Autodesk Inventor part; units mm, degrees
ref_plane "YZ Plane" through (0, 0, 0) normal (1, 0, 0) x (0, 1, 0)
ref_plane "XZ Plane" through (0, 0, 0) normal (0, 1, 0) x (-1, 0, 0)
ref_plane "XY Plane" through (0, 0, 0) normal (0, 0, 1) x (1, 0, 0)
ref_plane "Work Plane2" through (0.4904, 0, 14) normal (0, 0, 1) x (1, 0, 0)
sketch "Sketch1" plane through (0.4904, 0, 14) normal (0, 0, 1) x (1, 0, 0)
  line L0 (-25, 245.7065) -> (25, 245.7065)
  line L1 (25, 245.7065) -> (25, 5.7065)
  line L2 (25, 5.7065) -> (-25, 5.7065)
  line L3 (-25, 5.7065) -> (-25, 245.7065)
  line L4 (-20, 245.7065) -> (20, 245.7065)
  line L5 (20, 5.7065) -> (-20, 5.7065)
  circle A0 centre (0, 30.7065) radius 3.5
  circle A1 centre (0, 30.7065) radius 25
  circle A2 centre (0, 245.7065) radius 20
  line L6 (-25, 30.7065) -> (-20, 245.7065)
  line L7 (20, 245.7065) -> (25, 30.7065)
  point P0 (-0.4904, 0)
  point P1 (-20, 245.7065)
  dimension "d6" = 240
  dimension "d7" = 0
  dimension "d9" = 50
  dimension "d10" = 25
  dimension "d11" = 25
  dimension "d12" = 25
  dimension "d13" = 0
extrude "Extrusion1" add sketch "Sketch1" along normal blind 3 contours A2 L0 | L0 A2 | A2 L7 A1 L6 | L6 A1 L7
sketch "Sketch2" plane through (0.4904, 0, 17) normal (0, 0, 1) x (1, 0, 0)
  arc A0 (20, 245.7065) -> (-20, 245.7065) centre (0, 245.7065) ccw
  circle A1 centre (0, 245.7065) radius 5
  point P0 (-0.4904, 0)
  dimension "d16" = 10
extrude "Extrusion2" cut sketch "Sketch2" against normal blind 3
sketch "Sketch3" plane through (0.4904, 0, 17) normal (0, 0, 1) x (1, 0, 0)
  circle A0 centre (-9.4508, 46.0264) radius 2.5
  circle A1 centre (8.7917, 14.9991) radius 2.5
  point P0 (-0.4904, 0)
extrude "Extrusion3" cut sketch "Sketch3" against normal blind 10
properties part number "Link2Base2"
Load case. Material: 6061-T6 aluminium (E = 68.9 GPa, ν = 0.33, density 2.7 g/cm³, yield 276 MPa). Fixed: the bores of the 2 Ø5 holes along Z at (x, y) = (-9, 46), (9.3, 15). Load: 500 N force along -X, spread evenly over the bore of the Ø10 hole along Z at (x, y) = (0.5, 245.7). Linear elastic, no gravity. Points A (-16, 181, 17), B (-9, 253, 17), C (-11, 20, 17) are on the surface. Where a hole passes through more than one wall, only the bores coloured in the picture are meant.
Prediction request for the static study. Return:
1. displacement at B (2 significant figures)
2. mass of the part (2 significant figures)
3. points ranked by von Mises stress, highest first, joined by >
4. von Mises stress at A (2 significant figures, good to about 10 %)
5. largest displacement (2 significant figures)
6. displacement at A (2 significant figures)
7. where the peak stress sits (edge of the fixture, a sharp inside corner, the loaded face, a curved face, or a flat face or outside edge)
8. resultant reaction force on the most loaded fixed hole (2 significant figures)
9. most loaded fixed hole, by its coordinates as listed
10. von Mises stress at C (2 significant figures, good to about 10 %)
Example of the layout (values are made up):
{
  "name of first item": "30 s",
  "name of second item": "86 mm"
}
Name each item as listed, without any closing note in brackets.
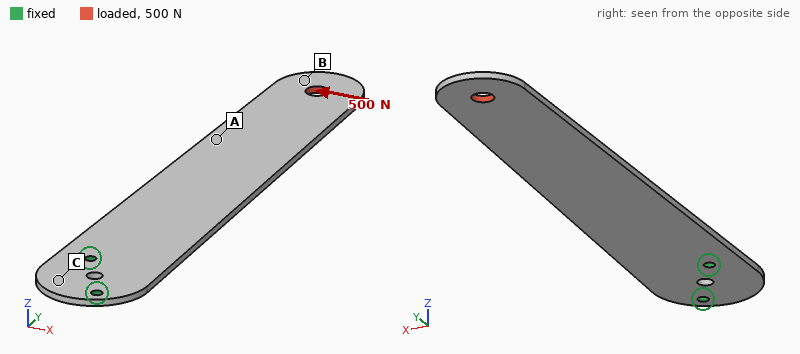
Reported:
{
  "displacement at B": "1.1 mm",
  "mass of the part": "90 g",
  "points ranked by von Mises stress, highest first, joined by >": "A > C > B",
  "von Mises stress at A": "27 MPa",
  "largest displacement": "1.2 mm",
  "displacement at A": "0.57 mm",
  "where the peak stress sits": "edge of the fixture",
  "resultant reaction force on the most loaded fixed hole": "3.0 kN",
  "most loaded fixed hole, by its coordinates as listed": "(-9, 46)",
  "von Mises stress at C": "16 MPa"
}
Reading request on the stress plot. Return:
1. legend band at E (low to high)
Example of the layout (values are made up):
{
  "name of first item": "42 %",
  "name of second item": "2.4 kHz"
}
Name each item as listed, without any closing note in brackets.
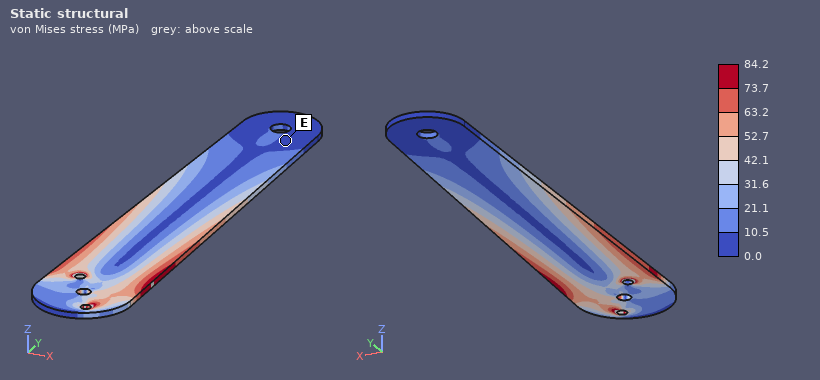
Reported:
{
  "legend band at E": "0.0 to 10.5 MPa"
}
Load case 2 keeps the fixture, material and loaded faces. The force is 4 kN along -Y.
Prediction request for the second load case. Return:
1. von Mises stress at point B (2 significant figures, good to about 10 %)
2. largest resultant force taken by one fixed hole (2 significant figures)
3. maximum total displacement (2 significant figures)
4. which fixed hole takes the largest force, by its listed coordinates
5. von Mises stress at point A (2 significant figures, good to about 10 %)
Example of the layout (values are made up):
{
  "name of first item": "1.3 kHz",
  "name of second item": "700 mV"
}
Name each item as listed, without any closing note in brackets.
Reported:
{
  "von Mises stress at point B": "22 MPa",
  "largest resultant force taken by one fixed hole": "2.6 kN",
  "maximum total displacement": "0.13 mm",
  "which fixed hole takes the largest force, by its listed coordinates": "(-9, 46)",
  "von Mises stress at point A": "31 MPa"
}
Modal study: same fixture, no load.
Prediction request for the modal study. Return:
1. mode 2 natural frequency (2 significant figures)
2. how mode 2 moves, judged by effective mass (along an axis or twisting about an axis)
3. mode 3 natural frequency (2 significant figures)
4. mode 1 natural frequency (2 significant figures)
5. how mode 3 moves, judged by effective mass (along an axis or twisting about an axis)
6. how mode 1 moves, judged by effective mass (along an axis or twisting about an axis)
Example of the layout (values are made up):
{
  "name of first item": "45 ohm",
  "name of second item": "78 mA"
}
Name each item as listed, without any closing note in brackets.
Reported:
{
  "mode 2 natural frequency": "330 Hz",
  "how mode 2 moves, judged by effective mass": "along Z",
  "mode 3 natural frequency": "520 Hz",
  "mode 1 natural frequency": "57 Hz",
  "how mode 3 moves, judged by effective mass": "twisting about Y",
  "how mode 1 moves, judged by effective mass": "along Z"
}
